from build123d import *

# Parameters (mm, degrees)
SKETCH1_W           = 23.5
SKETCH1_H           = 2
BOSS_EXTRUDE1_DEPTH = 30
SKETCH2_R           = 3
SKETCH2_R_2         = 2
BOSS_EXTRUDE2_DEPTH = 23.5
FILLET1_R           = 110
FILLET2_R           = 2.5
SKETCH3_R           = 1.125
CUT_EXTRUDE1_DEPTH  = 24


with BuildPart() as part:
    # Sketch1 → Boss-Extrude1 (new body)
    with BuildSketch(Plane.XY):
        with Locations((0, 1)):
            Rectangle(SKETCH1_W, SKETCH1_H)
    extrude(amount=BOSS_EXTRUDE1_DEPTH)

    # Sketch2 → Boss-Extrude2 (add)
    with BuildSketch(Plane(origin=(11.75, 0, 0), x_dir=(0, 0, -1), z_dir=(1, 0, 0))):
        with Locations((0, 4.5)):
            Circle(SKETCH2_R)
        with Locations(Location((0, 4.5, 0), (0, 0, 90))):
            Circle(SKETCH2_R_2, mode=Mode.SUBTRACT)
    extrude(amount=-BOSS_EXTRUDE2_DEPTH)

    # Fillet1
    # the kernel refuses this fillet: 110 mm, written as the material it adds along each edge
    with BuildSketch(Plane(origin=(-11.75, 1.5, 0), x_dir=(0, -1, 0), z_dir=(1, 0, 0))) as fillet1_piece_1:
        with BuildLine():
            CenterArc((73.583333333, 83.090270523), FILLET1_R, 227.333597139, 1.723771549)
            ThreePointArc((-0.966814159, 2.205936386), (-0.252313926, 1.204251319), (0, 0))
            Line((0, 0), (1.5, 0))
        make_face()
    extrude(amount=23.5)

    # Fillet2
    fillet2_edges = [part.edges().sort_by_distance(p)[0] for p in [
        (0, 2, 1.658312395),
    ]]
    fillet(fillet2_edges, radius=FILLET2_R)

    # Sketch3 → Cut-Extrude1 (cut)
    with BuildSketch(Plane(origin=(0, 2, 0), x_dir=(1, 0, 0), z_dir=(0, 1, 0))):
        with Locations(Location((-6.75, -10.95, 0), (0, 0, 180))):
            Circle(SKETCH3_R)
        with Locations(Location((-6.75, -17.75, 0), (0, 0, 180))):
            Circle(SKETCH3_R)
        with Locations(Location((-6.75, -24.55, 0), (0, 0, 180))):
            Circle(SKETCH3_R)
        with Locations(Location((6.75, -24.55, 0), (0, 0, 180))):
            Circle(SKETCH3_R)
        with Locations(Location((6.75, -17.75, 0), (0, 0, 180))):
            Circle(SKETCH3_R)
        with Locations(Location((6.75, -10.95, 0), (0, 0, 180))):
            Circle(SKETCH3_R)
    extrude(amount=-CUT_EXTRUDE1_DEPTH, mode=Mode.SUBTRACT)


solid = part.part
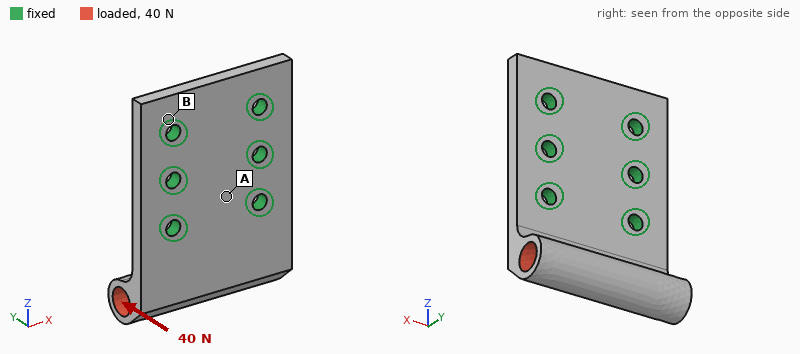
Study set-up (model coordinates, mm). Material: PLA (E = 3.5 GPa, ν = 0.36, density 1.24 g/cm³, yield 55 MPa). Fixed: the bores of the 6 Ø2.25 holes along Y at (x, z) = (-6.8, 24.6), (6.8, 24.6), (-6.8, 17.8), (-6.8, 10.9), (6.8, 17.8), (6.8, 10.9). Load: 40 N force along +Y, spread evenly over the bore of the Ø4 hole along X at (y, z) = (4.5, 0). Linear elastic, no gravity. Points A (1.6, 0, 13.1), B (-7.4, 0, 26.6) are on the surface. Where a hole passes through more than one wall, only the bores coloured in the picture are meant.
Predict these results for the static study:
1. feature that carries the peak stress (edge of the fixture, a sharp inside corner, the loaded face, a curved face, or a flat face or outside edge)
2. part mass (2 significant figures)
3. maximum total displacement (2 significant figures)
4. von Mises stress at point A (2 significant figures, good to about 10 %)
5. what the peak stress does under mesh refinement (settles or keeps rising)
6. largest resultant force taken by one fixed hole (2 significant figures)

edge of the fixture
2.2 g
0.43 mm
5.7 MPa
keeps rising
29 N
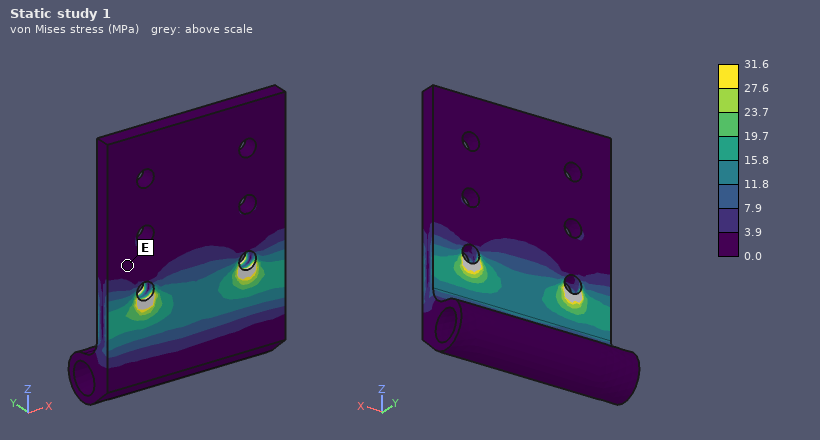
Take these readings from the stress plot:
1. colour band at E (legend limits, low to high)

0.0 to 3.9 MPa
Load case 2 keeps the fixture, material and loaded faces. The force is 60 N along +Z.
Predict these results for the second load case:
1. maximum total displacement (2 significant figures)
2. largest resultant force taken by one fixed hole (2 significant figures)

0.30 mm
23 N
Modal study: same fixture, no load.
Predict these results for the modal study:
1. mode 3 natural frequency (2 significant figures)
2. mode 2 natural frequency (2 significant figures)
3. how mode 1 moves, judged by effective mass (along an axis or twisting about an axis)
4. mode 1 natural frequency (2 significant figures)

10 kHz
4800 Hz
along Y
2100 Hz
